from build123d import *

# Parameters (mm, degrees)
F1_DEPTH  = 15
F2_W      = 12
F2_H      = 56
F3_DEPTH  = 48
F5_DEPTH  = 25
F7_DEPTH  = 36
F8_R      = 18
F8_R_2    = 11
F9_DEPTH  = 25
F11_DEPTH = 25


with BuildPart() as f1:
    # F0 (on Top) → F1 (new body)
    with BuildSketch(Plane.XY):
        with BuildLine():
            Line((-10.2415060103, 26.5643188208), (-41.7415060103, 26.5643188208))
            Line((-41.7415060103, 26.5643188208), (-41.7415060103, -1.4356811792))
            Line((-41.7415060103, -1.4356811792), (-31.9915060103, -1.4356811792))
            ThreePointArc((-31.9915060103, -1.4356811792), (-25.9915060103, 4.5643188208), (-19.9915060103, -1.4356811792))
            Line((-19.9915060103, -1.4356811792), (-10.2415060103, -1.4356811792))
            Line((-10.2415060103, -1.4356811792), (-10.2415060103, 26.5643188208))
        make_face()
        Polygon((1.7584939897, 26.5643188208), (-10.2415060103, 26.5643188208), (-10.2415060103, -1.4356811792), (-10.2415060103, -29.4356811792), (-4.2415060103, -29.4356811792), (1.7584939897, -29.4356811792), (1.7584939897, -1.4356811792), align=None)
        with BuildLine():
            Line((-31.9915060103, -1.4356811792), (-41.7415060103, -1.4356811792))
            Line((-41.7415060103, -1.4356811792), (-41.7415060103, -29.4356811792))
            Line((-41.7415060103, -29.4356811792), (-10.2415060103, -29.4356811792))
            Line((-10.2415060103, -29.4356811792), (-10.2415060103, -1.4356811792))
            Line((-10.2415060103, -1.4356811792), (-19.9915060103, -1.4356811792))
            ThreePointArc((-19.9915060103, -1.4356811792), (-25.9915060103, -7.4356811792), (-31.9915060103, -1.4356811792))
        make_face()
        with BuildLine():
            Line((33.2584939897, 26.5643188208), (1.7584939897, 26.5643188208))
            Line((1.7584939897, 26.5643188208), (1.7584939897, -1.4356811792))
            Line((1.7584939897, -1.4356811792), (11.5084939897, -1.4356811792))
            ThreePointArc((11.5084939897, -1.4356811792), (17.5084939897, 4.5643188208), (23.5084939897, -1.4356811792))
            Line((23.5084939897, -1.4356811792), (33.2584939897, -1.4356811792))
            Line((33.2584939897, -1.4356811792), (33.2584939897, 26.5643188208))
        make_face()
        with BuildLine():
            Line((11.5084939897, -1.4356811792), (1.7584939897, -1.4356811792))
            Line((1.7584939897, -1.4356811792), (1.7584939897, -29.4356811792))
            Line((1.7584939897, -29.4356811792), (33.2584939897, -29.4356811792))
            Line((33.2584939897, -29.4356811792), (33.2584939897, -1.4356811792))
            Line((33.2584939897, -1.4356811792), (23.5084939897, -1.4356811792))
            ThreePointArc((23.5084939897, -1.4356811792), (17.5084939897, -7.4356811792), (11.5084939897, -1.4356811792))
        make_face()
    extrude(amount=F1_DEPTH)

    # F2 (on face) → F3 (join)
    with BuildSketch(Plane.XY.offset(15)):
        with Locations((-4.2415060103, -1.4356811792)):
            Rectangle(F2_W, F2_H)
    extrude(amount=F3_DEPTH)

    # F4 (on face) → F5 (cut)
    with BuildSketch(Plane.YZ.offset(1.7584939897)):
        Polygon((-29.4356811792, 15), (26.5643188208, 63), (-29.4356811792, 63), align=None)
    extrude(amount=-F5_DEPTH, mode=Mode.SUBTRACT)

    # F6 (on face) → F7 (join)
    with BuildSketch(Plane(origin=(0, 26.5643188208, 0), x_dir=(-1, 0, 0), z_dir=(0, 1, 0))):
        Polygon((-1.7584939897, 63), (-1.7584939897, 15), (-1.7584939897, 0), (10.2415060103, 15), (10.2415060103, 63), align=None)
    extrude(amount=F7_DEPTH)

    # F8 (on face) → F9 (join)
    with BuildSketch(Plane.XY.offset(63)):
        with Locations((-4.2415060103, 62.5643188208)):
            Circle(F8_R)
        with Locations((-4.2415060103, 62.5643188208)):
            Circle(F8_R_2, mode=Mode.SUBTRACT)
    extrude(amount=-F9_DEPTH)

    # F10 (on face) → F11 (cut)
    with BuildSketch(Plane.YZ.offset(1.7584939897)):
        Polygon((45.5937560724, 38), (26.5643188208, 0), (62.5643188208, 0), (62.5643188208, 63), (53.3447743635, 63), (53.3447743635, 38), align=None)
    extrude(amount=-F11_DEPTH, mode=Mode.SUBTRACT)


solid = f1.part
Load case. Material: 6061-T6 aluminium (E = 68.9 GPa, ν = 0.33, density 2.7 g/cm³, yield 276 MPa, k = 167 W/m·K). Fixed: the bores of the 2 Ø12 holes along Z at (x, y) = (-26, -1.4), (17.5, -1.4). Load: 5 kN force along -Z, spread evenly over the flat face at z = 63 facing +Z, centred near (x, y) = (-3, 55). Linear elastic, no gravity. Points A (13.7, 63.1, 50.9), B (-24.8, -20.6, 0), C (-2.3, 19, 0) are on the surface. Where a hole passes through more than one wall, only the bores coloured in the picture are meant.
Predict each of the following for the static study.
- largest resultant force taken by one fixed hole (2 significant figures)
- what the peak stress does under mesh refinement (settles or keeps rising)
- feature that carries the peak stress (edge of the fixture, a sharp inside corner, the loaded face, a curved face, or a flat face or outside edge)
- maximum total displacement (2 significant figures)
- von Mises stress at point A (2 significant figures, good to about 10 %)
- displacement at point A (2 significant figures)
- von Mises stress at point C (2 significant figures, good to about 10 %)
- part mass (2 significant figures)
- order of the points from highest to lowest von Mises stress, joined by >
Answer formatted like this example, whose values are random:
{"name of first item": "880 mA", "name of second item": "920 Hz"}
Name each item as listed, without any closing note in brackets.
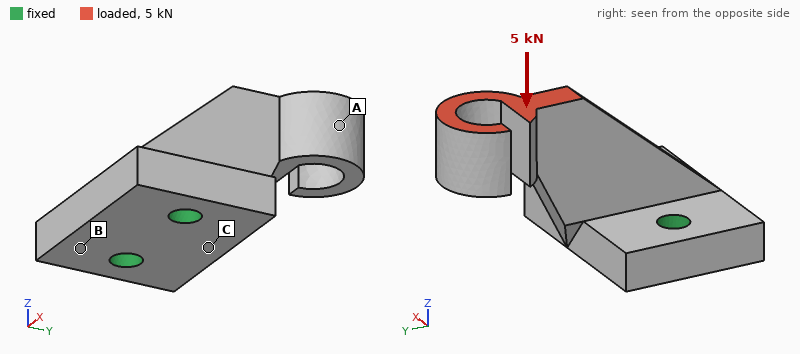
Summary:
{"largest resultant force taken by one fixed hole": "3.0 kN", "what the peak stress does under mesh refinement": "keeps rising", "feature that carries the peak stress": "a sharp inside corner", "maximum total displacement": "0.70 mm", "von Mises stress at point A": "100 MPa", "displacement at point A": "0.27 mm", "von Mises stress at point C": "54 MPa", "part mass": "270 g", "order of the points from highest to lowest von Mises stress, joined by >": "A > C > B"}
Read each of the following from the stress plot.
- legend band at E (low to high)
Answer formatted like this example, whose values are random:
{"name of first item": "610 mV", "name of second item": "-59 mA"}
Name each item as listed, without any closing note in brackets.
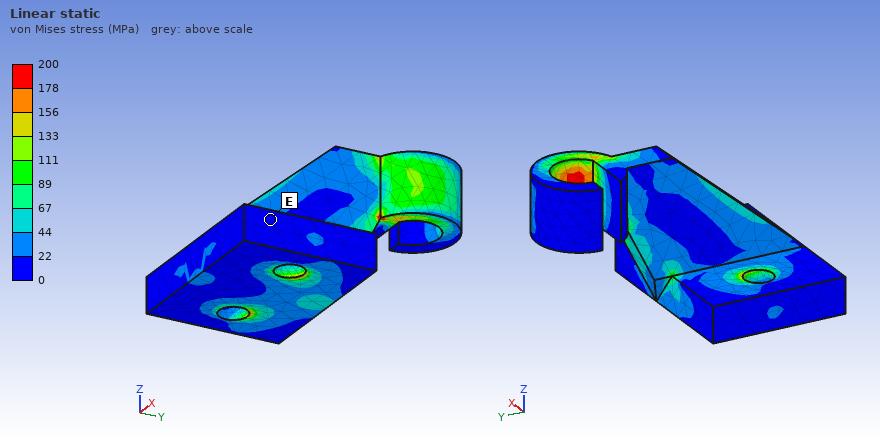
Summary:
{"legend band at E": "0 to 22 MPa"}
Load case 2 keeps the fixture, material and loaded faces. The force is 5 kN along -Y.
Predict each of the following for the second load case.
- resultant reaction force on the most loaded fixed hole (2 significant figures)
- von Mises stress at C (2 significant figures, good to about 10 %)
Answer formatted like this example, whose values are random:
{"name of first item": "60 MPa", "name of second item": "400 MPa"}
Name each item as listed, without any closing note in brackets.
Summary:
{"resultant reaction force on the most loaded fixed hole": "2.7 kN", "von Mises stress at C": "45 MPa"}
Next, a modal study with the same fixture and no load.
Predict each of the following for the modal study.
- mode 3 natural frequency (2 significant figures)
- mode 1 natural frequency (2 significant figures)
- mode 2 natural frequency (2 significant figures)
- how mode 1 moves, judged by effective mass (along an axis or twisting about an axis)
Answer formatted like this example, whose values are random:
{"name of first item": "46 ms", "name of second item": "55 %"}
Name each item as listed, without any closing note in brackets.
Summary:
{"mode 3 natural frequency": "2600 Hz", "mode 1 natural frequency": "1300 Hz", "mode 2 natural frequency": "2100 Hz", "how mode 1 moves, judged by effective mass": "along X"}
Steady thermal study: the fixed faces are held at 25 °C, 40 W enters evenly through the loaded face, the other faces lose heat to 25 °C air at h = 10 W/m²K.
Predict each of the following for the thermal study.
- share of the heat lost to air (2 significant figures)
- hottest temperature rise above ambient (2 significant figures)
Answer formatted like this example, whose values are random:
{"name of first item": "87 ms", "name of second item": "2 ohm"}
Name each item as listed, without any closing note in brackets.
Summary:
{"share of the heat lost to air": "7.4 %", "hottest temperature rise above ambient": "56 K"}
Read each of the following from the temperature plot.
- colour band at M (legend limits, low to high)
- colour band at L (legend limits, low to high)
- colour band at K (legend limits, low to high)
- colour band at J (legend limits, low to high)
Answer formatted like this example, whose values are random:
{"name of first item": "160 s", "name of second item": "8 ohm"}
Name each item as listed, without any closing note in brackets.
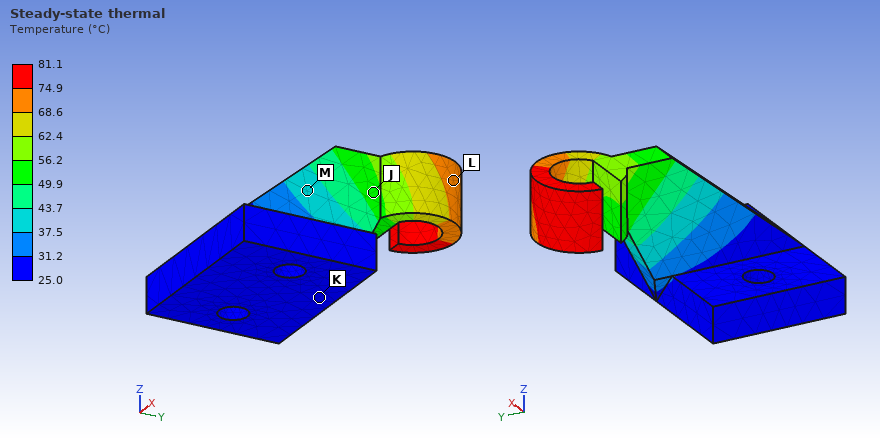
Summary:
{"colour band at M": "37.5 to 43.7 °C", "colour band at L": "68.6 to 74.9 °C", "colour band at K": "25.0 to 31.2 °C", "colour band at J": "49.9 to 56.2 °C"}
